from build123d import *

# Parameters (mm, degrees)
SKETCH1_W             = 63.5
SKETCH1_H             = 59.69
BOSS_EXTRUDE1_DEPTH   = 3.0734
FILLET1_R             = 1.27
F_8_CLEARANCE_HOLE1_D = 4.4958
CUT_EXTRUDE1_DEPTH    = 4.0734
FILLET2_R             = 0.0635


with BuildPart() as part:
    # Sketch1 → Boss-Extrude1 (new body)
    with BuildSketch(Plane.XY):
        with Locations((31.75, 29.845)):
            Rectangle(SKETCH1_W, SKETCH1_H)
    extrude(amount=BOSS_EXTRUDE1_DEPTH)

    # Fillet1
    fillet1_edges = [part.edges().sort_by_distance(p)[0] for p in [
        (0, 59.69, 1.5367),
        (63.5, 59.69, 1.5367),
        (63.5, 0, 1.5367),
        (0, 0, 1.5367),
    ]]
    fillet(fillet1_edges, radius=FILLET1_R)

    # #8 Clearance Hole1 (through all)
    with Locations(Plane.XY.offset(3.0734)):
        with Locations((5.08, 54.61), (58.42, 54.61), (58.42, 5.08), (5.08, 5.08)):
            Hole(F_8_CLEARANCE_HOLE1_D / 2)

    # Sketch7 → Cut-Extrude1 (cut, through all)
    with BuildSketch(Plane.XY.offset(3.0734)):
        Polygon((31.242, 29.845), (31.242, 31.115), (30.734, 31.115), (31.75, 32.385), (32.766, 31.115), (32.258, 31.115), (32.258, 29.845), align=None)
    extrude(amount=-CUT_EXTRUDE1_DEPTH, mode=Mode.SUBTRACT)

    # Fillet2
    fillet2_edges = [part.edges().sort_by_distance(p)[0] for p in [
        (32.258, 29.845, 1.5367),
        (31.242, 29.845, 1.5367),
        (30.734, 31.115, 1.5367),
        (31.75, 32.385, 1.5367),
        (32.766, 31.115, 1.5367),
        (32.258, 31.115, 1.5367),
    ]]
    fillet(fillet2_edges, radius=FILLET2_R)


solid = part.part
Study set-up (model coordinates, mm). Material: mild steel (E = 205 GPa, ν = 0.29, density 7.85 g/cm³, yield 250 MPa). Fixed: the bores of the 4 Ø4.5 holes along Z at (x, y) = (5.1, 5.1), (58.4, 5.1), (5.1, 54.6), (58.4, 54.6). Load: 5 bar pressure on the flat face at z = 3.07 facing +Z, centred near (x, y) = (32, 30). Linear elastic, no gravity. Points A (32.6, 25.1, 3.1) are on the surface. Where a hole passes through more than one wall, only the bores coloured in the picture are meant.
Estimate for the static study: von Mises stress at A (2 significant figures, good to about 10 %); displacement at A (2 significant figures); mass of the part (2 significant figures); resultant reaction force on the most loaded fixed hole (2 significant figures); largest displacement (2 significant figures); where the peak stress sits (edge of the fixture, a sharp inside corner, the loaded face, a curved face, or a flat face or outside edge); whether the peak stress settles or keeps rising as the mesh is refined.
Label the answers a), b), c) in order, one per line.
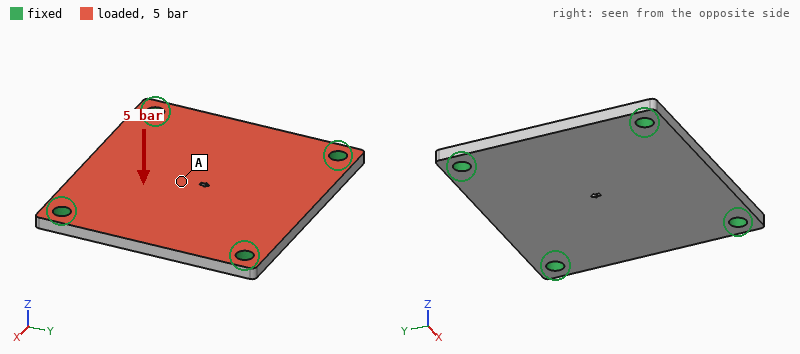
a) 42 MPa
b) 44 µm
c) 90 g
d) 470 N
e) 45 µm
f) edge of the fixture
g) keeps rising
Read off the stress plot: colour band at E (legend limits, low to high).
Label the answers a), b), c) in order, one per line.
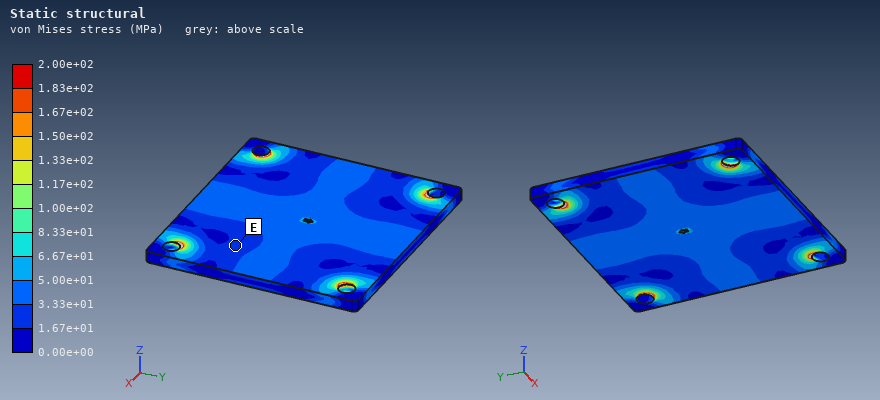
a) 1.67e+01 to 3.33e+01 MPa
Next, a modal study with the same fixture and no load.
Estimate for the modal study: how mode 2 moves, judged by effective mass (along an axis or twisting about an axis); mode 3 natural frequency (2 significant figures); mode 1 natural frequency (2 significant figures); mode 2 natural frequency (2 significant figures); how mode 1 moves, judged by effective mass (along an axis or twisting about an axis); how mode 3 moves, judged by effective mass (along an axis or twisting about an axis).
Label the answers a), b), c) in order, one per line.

a) twisting about X
b) 7400 Hz
c) 4200 Hz
d) 6700 Hz
e) along Z
f) twisting about Y
